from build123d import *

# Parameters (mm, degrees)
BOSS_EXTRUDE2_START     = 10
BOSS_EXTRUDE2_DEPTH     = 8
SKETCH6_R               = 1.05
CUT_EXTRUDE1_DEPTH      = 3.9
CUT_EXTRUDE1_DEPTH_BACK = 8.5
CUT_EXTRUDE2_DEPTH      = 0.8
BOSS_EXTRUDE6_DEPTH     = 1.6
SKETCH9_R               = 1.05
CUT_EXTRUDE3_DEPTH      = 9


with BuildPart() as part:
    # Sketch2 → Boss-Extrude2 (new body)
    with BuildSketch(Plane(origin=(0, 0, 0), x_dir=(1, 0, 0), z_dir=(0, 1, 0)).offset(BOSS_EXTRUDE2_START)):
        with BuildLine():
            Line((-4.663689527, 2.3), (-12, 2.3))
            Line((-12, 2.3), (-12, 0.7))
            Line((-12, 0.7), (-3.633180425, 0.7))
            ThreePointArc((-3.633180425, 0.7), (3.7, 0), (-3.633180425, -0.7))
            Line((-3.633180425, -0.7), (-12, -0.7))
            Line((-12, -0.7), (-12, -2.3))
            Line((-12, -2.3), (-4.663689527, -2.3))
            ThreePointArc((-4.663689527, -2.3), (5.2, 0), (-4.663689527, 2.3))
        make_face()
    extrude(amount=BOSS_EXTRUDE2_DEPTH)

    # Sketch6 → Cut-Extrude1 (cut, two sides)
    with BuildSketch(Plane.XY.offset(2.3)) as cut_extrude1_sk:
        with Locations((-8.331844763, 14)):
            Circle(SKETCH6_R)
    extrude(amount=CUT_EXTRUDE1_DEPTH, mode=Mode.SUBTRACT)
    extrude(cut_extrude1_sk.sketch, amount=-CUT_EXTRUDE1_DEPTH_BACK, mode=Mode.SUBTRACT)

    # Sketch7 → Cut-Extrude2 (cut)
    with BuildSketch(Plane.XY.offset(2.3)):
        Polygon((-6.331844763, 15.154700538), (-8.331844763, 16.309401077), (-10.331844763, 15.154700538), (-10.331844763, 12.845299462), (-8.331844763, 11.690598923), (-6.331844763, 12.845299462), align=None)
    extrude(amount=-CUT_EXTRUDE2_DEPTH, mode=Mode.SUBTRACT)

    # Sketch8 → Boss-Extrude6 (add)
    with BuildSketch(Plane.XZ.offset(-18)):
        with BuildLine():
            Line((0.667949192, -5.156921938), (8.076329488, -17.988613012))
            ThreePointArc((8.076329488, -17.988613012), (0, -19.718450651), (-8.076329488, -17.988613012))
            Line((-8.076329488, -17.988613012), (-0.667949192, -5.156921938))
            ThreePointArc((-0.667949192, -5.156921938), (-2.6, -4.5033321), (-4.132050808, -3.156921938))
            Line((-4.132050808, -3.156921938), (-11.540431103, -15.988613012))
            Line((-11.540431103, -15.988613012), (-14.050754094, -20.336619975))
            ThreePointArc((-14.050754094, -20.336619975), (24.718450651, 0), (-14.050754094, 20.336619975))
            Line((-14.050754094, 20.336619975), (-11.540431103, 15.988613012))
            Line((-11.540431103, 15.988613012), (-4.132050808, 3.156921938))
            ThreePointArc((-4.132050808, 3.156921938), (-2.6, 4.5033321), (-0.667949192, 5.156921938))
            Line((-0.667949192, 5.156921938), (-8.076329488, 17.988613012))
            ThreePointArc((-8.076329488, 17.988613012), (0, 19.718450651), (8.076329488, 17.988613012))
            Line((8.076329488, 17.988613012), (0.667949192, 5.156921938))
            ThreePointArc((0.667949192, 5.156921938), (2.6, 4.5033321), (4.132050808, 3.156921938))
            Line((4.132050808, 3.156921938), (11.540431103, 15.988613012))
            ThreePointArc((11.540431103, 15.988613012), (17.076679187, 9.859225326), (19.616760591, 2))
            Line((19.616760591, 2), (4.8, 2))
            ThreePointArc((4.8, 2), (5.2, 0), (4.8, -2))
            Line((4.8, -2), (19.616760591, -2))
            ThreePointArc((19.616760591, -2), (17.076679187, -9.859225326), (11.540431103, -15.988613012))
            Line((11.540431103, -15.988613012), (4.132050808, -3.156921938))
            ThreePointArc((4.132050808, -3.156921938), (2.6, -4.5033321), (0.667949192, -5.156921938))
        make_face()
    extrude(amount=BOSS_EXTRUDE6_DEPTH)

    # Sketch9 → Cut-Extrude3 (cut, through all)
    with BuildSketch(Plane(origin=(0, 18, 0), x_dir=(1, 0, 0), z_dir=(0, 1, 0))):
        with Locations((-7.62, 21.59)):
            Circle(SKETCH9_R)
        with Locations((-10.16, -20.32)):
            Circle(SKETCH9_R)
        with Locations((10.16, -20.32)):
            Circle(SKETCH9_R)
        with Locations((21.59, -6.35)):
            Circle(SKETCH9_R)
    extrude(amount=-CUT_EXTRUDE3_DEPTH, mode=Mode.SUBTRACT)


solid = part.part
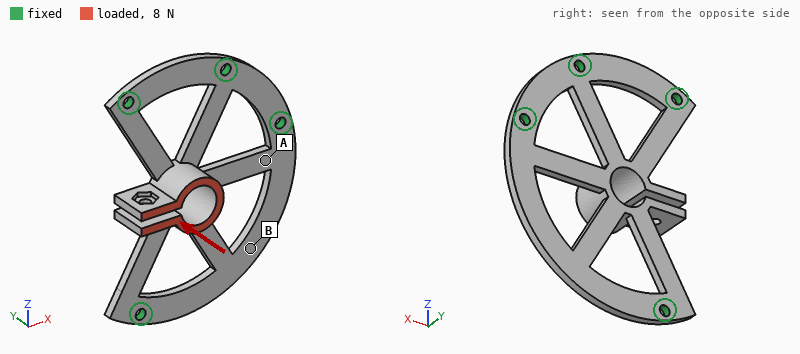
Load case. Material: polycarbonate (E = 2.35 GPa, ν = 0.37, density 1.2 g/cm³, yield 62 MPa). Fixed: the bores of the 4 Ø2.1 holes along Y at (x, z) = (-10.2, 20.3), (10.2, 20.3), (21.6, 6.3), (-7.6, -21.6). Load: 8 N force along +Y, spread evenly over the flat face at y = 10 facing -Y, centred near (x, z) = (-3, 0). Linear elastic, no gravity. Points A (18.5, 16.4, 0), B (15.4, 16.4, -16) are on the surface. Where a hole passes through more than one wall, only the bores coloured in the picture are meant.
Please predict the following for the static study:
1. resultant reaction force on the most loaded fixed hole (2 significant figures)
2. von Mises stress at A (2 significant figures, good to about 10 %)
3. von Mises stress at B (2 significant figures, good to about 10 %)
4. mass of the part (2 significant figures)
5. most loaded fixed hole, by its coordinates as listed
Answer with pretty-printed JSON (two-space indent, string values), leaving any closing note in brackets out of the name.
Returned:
{
  "resultant reaction force on the most loaded fixed hole": "3.6 N",
  "von Mises stress at A": "3.4 MPa",
  "von Mises stress at B": "1.2 MPa",
  "mass of the part": "2.0 g",
  "most loaded fixed hole, by its coordinates as listed": "(-7.6, -21.6)"
}
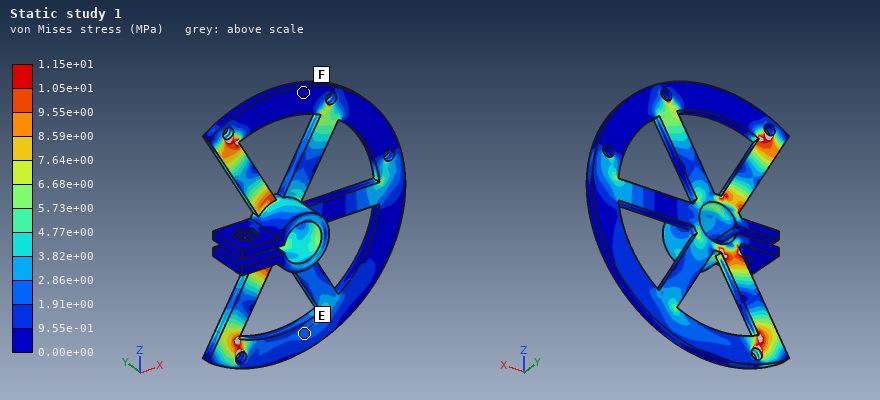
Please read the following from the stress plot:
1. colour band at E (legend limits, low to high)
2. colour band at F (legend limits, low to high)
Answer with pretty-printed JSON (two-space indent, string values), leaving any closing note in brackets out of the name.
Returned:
{
  "colour band at E": "1.91e+00 to 2.86e+00 MPa",
  "colour band at F": "0.00e+00 to 9.55e-01 MPa"
}
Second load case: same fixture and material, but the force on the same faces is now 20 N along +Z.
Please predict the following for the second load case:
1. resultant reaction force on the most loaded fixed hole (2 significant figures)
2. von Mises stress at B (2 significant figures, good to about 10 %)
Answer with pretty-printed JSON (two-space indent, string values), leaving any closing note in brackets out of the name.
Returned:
{
  "resultant reaction force on the most loaded fixed hole": "8.4 N",
  "von Mises stress at B": "2.7 MPa"
}
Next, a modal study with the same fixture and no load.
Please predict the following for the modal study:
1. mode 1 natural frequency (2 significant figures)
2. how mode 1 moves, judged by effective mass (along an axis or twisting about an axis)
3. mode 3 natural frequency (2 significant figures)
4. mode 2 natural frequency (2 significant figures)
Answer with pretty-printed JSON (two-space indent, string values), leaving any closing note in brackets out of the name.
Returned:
{
  "mode 1 natural frequency": "770 Hz",
  "how mode 1 moves, judged by effective mass": "along Y",
  "mode 3 natural frequency": "1600 Hz",
  "mode 2 natural frequency": "910 Hz"
}
